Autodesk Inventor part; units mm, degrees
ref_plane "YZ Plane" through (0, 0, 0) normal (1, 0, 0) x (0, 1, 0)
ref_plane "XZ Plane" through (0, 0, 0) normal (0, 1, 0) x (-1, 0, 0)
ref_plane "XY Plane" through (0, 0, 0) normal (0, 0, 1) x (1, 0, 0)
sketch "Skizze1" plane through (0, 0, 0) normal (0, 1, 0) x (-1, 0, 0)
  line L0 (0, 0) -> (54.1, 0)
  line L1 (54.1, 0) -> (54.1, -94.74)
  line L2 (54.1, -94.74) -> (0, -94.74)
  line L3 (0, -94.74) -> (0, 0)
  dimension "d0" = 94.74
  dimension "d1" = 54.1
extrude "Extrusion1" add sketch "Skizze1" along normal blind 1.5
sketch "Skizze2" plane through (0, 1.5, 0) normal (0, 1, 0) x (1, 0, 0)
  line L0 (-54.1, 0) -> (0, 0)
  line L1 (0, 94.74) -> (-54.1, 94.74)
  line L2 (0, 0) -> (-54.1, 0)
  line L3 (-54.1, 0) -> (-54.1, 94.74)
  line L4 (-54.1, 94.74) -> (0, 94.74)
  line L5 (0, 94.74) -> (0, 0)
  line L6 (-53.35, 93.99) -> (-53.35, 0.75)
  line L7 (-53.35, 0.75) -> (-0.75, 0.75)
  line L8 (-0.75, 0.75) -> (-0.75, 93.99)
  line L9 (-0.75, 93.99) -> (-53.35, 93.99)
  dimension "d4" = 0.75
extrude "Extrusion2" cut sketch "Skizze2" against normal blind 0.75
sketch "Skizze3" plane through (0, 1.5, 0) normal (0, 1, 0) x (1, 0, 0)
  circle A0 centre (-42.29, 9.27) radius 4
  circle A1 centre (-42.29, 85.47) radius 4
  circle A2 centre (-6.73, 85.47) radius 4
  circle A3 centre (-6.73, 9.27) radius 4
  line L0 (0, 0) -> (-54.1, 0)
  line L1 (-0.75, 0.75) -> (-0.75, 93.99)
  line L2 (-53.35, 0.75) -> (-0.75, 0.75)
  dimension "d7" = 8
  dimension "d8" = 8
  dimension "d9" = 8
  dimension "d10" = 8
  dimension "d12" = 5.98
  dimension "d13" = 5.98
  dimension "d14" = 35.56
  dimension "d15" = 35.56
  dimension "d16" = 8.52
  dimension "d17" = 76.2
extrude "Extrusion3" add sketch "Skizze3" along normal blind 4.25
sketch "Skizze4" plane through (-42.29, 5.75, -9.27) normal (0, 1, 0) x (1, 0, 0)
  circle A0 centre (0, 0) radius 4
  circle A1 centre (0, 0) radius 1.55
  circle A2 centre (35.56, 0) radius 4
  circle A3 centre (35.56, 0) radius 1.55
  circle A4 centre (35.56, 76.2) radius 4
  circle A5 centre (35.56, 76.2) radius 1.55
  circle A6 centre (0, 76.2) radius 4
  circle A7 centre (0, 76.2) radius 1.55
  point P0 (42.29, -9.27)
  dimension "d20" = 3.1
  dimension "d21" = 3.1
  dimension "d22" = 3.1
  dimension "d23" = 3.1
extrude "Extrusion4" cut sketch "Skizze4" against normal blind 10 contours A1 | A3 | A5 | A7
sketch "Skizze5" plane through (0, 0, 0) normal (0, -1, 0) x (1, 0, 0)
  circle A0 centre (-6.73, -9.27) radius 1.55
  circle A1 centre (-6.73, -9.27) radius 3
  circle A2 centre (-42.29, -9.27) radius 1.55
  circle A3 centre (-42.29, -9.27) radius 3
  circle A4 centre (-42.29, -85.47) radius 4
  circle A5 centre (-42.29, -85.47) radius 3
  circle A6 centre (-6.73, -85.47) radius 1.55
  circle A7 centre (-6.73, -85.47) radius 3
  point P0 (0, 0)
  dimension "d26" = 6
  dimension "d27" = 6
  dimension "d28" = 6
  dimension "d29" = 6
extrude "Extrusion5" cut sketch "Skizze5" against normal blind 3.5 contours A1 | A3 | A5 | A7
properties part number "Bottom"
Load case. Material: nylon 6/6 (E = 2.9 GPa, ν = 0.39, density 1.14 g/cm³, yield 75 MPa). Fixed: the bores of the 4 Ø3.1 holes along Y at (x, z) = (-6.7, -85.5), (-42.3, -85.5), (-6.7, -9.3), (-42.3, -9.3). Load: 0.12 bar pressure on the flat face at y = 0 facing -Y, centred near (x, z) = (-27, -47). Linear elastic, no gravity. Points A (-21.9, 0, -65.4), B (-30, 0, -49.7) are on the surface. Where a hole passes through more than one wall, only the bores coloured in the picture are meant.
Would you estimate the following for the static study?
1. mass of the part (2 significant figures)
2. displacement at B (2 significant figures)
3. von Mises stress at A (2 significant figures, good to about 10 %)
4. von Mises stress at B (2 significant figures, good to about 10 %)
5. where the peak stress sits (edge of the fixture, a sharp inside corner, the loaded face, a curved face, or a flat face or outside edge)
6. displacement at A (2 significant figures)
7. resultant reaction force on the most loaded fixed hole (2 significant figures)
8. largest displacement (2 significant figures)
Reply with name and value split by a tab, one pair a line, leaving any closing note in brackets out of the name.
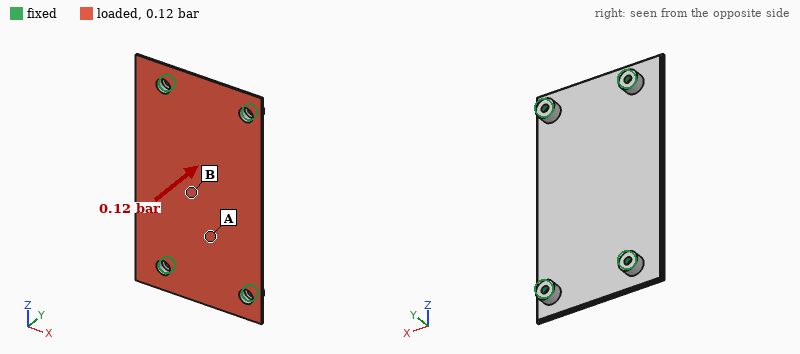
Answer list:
mass of the part	9.0 g
displacement at B	1.1 mm
von Mises stress at A	2.7 MPa
von Mises stress at B	6.9 MPa
where the peak stress sits	a curved face
displacement at A	0.73 mm
resultant reaction force on the most loaded fixed hole	28 N
largest displacement	1.3 mm
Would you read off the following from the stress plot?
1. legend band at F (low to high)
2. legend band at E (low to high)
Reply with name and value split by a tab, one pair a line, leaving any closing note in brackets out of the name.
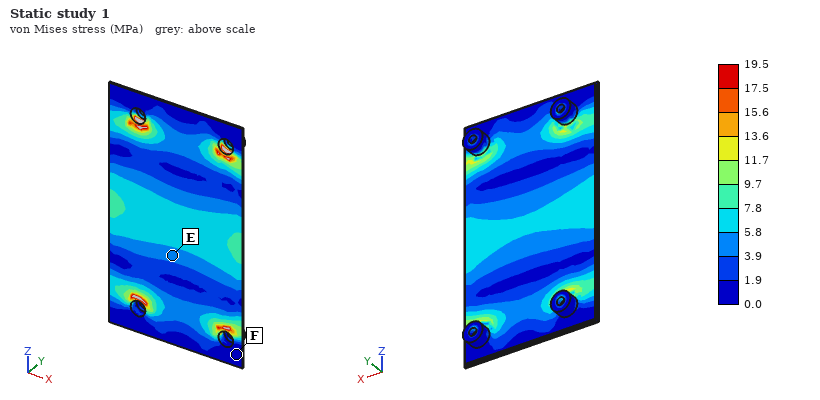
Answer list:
legend band at F	0.0 to 1.9 MPa
legend band at E	3.9 to 5.8 MPa
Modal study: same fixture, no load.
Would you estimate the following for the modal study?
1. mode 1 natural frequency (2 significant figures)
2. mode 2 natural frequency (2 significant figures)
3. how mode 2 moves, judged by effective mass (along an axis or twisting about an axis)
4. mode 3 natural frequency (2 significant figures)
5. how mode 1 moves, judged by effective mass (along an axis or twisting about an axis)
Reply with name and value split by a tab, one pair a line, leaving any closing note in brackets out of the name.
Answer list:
mode 1 natural frequency	440 Hz
mode 2 natural frequency	610 Hz
how mode 2 moves, judged by effective mass	twisting about Z
mode 3 natural frequency	1200 Hz
how mode 1 moves, judged by effective mass	along Y
